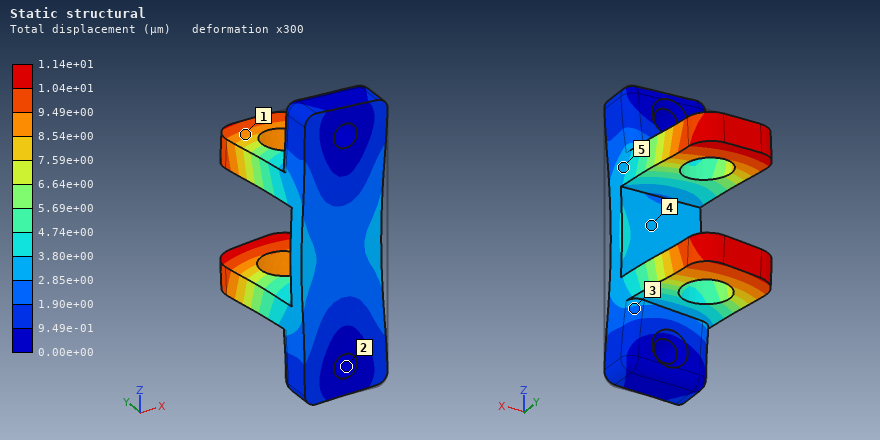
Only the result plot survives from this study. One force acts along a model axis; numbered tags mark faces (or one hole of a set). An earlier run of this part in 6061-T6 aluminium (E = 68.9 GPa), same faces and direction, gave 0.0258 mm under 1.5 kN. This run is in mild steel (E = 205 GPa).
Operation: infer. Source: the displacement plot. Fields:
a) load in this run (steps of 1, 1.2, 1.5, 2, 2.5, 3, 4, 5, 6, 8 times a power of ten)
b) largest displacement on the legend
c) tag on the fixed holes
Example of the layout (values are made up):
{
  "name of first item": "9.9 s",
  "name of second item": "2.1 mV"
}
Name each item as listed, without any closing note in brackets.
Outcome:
{
  "load in this run": "2 kN",
  "largest displacement on the legend": "1.14e+01 µm",
  "tag on the fixed holes": "2"
}
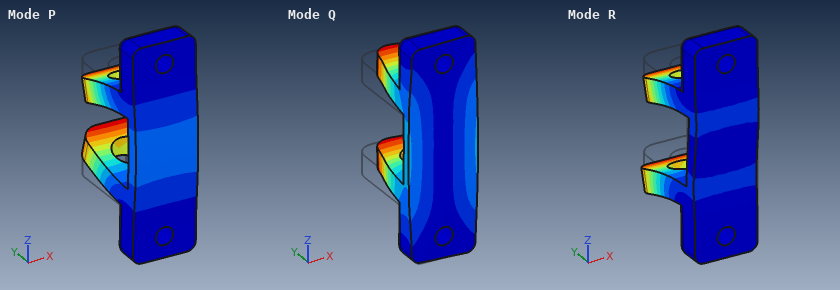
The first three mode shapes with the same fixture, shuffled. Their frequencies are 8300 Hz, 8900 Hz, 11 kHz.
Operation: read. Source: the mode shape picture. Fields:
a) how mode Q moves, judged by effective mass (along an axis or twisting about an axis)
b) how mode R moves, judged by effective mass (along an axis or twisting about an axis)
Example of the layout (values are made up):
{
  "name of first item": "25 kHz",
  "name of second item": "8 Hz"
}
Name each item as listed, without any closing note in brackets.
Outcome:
{
  "how mode Q moves, judged by effective mass": "along X",
  "how mode R moves, judged by effective mass": "along Z"
}
